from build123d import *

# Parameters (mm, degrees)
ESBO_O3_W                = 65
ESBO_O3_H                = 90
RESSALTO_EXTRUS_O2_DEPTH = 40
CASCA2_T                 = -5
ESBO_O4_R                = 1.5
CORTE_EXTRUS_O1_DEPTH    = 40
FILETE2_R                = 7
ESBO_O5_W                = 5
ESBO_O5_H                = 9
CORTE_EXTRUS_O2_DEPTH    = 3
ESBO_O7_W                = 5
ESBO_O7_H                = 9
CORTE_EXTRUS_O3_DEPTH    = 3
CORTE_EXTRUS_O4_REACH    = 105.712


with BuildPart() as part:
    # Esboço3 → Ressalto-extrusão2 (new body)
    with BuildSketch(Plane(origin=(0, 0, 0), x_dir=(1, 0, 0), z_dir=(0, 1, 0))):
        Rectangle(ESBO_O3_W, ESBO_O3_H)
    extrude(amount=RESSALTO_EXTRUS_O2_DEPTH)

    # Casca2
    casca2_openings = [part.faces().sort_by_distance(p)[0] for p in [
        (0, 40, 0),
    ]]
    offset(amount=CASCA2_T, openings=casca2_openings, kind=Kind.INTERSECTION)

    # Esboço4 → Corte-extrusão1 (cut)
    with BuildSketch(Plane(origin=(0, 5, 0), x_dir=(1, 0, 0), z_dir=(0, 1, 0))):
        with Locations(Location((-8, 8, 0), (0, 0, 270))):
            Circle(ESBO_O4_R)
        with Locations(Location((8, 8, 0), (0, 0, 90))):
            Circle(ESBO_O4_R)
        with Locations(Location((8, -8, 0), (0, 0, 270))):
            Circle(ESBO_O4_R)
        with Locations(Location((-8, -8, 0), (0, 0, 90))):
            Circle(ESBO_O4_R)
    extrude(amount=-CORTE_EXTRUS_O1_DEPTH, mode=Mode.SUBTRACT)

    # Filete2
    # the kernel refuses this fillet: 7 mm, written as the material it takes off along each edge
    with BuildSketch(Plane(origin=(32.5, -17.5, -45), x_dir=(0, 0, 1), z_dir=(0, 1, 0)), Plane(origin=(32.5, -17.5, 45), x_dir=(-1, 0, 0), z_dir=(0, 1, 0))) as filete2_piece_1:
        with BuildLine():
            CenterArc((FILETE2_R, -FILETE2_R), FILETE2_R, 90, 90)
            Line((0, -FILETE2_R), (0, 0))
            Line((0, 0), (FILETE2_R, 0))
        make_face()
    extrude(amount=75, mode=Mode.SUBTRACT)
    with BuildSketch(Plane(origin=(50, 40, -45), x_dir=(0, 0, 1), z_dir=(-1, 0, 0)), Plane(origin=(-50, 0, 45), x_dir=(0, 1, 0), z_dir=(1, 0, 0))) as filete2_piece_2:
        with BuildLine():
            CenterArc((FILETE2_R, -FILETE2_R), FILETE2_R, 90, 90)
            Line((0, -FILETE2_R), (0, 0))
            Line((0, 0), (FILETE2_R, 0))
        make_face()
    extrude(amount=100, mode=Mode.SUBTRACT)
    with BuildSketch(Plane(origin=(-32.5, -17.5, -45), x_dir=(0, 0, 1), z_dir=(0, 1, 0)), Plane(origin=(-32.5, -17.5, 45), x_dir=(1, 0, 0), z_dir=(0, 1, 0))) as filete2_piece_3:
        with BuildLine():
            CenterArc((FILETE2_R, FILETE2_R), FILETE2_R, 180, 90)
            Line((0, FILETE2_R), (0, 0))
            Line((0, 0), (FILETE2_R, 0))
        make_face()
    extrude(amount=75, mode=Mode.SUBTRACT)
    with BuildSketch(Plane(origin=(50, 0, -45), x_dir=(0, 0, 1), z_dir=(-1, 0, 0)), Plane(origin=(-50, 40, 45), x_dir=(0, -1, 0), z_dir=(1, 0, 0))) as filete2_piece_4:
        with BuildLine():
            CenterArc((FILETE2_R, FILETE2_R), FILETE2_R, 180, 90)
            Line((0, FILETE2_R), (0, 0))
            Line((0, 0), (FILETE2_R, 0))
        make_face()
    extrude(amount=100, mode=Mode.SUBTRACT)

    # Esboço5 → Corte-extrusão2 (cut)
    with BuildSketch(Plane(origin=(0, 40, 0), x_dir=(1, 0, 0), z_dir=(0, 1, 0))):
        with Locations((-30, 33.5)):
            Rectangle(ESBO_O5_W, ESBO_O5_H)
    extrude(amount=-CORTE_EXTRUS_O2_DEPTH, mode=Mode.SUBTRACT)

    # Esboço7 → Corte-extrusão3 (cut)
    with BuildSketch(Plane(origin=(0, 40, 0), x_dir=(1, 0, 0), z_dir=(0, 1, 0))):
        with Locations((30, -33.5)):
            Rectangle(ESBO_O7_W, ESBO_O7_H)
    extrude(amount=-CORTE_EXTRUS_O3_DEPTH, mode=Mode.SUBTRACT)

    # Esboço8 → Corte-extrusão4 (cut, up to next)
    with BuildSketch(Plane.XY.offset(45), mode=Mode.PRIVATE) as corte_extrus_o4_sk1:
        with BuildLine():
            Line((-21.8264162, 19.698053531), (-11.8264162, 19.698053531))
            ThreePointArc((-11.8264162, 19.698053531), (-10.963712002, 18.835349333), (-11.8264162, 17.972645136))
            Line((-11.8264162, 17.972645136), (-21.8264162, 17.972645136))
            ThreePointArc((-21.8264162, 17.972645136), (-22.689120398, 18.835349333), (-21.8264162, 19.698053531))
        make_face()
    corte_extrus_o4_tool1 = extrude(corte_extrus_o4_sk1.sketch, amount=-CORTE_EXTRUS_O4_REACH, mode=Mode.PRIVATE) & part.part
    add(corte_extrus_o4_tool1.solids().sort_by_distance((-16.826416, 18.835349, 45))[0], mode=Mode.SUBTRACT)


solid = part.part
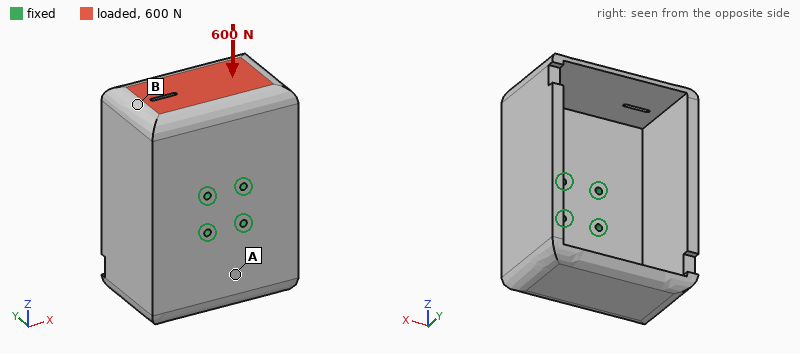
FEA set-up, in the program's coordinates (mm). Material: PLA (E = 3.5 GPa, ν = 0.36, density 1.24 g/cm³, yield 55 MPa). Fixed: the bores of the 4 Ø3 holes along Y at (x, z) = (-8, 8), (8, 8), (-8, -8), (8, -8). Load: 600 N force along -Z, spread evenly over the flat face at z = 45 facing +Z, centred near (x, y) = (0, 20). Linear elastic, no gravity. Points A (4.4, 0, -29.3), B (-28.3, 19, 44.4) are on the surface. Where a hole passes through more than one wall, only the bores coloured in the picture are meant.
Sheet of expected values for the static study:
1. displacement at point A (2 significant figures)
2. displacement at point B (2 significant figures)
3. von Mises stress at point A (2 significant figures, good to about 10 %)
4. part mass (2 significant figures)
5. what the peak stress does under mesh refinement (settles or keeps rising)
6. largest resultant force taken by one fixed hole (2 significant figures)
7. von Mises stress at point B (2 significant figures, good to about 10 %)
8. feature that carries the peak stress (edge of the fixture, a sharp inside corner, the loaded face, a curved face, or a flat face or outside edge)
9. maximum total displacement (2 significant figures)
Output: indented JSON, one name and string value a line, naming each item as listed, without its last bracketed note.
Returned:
{
  "displacement at point A": "0.31 mm",
  "displacement at point B": "0.68 mm",
  "von Mises stress at point A": "3.5 MPa",
  "part mass": "93 g",
  "what the peak stress does under mesh refinement": "keeps rising",
  "largest resultant force taken by one fixed hole": "280 N",
  "von Mises stress at point B": "7.3 MPa",
  "feature that carries the peak stress": "edge of the fixture",
  "maximum total displacement": "1.2 mm"
}
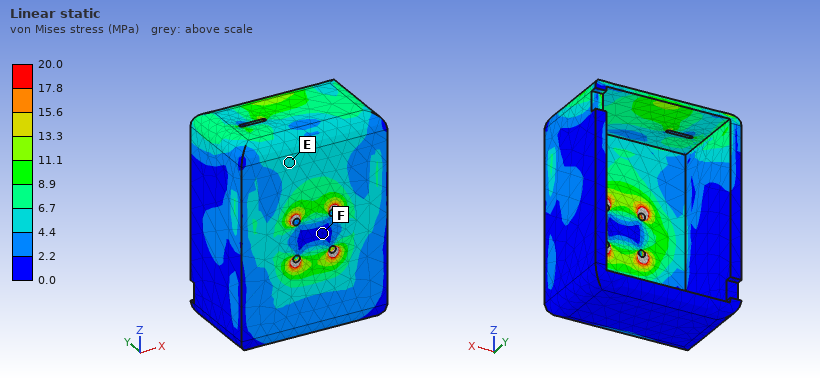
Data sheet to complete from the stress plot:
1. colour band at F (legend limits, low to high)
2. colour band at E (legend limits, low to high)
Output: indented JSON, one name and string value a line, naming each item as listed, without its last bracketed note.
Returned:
{
  "colour band at F": "0.0 to 2.2 MPa",
  "colour band at E": "4.4 to 6.7 MPa"
}
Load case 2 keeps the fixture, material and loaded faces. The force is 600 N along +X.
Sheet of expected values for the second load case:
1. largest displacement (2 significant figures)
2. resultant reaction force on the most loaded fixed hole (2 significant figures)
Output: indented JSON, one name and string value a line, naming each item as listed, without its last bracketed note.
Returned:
{
  "largest displacement": "1.4 mm",
  "resultant reaction force on the most loaded fixed hole": "760 N"
}
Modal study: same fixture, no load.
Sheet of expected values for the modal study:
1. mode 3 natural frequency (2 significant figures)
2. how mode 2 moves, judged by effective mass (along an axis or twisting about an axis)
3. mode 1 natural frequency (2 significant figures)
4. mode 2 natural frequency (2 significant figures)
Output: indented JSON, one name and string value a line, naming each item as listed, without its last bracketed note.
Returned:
{
  "mode 3 natural frequency": "630 Hz",
  "how mode 2 moves, judged by effective mass": "along X",
  "mode 1 natural frequency": "440 Hz",
  "mode 2 natural frequency": "520 Hz"
}
